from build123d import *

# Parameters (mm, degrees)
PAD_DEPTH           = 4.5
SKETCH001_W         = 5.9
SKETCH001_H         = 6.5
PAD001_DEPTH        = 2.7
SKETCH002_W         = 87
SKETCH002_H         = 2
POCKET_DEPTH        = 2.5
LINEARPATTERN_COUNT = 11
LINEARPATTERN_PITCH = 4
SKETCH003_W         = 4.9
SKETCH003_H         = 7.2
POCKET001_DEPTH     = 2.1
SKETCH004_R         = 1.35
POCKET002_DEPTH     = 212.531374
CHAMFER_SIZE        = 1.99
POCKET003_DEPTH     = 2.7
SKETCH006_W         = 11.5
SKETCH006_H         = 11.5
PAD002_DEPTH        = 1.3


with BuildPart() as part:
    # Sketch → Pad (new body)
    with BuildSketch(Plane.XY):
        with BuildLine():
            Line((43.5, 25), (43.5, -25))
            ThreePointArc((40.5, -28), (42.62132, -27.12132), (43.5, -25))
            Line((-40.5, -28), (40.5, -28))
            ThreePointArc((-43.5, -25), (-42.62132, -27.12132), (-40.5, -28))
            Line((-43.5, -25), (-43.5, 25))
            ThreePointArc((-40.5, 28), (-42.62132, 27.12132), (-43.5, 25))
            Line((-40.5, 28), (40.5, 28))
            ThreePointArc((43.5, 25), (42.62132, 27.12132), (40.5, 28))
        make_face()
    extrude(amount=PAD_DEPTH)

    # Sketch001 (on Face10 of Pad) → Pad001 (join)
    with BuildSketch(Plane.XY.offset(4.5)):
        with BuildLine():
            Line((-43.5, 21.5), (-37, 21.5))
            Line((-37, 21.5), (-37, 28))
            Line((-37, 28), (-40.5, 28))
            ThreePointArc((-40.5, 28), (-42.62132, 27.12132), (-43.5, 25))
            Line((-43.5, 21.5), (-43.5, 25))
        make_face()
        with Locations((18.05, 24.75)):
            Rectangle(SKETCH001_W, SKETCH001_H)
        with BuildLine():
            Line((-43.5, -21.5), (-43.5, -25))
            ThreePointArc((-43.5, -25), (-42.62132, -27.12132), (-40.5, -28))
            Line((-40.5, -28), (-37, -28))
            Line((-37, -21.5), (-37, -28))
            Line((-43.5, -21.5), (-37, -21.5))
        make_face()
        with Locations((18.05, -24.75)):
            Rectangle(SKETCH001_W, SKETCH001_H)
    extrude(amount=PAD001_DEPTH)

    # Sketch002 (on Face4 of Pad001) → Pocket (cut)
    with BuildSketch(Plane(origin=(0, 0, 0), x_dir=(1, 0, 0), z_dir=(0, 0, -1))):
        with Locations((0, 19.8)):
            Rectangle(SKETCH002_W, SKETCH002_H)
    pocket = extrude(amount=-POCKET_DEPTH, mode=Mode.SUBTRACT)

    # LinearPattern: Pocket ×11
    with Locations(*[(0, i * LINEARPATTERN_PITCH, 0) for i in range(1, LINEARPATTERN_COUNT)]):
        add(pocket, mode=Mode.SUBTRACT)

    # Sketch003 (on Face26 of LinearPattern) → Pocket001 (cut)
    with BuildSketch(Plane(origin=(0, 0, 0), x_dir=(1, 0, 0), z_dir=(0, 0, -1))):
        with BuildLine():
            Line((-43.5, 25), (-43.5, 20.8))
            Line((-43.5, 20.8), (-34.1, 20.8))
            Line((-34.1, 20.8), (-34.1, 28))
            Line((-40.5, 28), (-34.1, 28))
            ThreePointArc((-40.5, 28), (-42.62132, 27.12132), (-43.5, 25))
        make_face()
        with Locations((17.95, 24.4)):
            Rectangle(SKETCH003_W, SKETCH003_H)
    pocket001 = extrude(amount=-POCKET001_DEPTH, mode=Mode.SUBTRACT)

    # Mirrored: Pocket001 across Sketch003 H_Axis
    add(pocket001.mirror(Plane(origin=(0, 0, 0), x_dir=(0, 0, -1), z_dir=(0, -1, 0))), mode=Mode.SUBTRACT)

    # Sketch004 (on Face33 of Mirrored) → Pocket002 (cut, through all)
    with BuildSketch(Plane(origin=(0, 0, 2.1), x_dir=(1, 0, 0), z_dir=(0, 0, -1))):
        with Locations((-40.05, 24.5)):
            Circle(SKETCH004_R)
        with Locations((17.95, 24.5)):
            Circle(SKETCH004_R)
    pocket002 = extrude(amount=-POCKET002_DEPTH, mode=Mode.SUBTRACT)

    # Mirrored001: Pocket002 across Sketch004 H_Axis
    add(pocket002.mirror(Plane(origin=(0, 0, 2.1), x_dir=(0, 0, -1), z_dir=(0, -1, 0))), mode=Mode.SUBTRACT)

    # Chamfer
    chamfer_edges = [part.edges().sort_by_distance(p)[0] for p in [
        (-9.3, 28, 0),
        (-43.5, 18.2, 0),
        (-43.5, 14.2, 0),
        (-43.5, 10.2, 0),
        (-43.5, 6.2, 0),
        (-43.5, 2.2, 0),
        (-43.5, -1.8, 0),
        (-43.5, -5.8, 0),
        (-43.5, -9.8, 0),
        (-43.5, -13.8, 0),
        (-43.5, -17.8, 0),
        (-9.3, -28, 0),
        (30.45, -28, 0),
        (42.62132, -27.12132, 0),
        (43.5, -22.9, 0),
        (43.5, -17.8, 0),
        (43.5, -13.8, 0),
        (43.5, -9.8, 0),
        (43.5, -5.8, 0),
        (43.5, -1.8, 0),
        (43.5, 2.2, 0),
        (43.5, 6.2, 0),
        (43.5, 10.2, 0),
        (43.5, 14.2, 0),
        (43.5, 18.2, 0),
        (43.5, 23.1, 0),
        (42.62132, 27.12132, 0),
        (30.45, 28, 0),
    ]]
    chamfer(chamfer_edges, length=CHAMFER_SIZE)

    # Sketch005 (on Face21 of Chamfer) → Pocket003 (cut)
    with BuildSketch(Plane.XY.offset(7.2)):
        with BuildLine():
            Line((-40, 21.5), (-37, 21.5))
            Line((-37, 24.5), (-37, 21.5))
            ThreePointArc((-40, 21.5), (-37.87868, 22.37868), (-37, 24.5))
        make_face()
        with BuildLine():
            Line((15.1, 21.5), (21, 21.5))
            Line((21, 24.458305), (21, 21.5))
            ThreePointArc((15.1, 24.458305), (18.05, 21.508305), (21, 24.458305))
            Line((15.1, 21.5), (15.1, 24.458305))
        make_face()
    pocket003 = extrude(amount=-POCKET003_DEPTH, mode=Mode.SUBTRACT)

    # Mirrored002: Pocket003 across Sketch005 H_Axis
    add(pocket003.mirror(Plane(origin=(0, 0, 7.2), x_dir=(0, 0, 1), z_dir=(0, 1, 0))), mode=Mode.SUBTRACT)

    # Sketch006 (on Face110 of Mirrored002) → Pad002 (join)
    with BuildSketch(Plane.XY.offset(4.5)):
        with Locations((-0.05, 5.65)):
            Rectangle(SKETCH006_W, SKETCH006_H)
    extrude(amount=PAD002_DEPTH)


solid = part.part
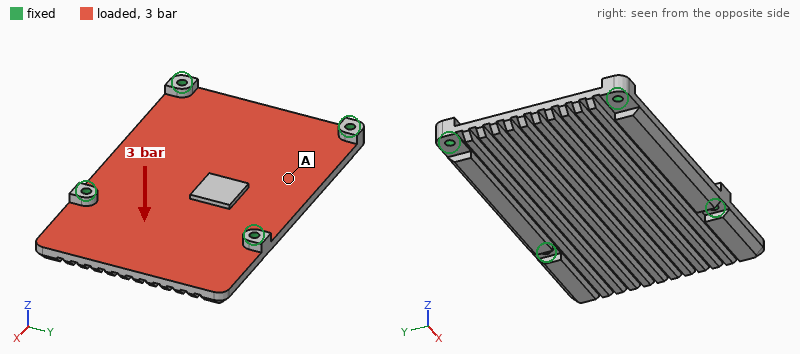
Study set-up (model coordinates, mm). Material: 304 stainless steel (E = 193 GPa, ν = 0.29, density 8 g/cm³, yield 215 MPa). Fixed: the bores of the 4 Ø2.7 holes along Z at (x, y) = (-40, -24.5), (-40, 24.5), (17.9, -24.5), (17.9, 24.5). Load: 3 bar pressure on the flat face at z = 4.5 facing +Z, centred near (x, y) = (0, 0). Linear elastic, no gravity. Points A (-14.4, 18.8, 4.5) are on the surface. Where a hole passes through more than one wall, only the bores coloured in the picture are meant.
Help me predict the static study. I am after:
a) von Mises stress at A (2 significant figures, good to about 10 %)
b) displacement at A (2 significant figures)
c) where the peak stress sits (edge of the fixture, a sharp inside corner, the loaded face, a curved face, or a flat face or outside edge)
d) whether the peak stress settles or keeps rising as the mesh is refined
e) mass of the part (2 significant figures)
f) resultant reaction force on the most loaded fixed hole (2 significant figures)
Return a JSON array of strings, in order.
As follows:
["20 MPa", "22 µm", "edge of the fixture", "keeps rising", "130 g", "490 N"]
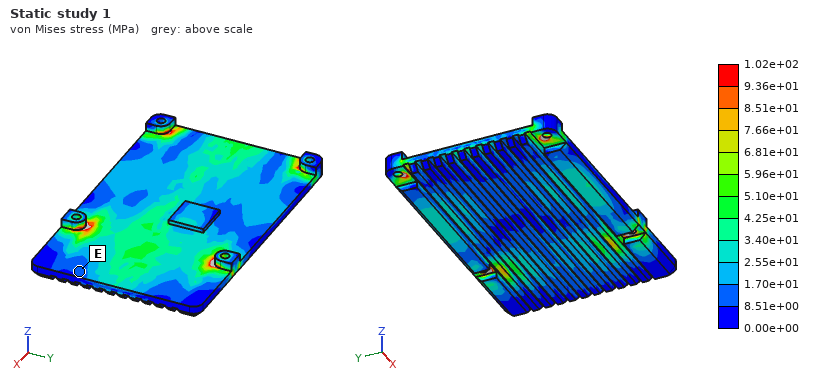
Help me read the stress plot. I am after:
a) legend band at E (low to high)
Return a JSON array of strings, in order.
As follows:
["8.51e+00 to 1.70e+01 MPa"]
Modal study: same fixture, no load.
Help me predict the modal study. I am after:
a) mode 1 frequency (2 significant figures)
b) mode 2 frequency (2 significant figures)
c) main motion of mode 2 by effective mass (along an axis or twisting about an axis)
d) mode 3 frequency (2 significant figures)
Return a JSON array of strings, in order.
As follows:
["2800 Hz", "3000 Hz", "along Z", "4700 Hz"]
